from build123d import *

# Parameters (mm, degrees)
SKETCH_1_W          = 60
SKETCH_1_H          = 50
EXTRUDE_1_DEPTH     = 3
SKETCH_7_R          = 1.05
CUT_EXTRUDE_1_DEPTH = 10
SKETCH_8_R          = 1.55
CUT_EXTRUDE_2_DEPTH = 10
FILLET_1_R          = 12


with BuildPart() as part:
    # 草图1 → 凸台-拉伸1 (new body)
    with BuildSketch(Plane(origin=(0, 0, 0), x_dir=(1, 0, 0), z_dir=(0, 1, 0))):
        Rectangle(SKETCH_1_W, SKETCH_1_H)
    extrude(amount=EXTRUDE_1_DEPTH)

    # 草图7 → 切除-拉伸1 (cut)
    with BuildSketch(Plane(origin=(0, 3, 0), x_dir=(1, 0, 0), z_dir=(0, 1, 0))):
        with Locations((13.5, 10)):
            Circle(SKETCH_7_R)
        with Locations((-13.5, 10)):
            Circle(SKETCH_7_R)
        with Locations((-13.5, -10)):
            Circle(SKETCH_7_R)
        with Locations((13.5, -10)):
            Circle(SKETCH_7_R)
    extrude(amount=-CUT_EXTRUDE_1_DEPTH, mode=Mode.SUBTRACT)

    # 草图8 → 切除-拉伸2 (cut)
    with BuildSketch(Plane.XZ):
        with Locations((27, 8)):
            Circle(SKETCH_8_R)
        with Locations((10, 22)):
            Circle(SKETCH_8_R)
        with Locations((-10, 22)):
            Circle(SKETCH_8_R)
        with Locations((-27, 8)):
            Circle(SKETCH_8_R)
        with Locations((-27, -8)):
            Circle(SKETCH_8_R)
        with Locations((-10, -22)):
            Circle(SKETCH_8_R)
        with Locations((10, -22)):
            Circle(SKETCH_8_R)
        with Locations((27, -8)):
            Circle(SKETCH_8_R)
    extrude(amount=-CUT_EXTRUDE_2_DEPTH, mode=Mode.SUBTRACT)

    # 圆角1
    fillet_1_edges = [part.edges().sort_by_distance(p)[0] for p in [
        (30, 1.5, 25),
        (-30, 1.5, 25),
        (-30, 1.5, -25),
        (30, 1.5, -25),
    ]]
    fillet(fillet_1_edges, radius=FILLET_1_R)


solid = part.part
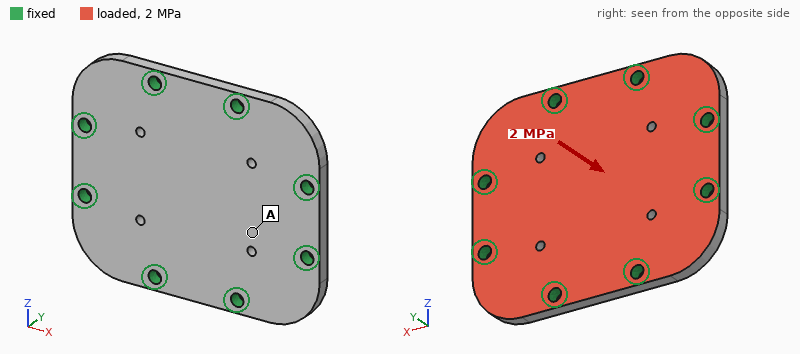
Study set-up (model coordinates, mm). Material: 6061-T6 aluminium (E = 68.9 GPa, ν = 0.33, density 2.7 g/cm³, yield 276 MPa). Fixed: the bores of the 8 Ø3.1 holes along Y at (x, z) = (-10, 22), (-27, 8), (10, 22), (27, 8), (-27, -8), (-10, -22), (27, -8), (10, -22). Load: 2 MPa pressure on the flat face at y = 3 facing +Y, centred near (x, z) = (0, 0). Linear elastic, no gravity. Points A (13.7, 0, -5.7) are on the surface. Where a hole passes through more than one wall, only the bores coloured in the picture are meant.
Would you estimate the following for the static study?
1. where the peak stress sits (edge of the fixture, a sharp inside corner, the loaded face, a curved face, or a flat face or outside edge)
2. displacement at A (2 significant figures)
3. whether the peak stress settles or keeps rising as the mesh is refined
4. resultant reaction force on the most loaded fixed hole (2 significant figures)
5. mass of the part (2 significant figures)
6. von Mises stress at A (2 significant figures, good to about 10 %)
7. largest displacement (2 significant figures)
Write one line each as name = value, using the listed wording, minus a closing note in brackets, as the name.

where the peak stress sits = edge of the fixture
displacement at A = 52 µm
whether the peak stress settles or keeps rising as the mesh is refined = keeps rising
resultant reaction force on the most loaded fixed hole = 780 N
mass of the part = 23 g
von Mises stress at A = 42 MPa
largest displacement = 93 µm
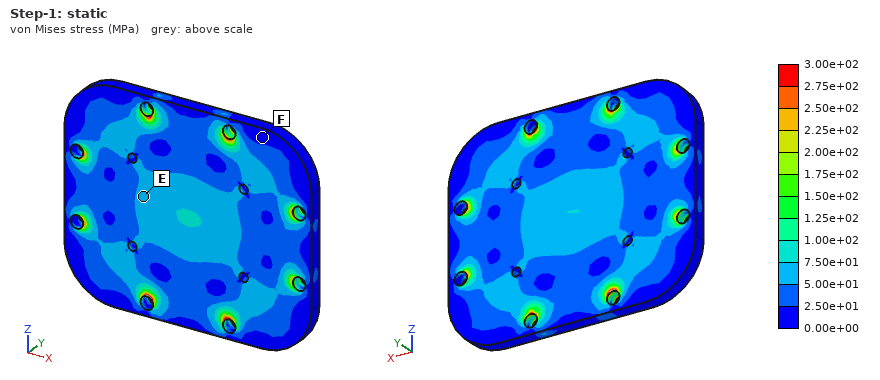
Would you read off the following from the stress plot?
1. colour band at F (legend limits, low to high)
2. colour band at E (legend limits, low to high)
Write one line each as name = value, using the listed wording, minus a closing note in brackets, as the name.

colour band at F = 0.00e+00 to 2.50e+01 MPa
colour band at E = 5.00e+01 to 7.50e+01 MPa
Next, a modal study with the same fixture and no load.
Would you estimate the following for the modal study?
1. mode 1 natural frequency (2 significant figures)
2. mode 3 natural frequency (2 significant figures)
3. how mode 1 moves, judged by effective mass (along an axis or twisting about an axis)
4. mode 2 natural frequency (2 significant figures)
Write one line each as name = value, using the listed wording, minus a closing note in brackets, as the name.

mode 1 natural frequency = 10000 Hz
mode 3 natural frequency = 21 kHz
how mode 1 moves, judged by effective mass = along Y
mode 2 natural frequency = 18 kHz
